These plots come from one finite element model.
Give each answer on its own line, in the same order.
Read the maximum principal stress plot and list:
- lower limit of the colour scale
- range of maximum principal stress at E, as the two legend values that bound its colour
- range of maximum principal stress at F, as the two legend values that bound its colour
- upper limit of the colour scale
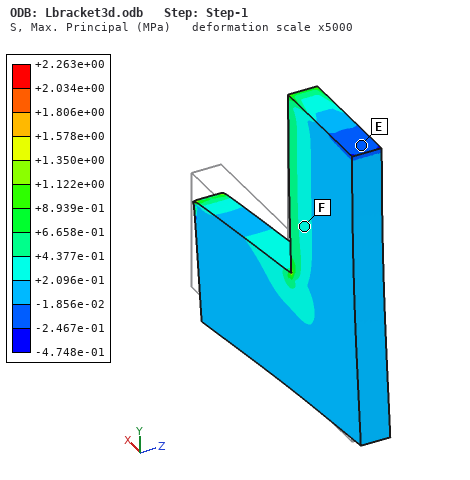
-4.748e-01 MPa
-2.467e-01 to -1.856e-02 MPa
+2.096e-01 to +4.377e-01 MPa
+2.263e+00 MPa
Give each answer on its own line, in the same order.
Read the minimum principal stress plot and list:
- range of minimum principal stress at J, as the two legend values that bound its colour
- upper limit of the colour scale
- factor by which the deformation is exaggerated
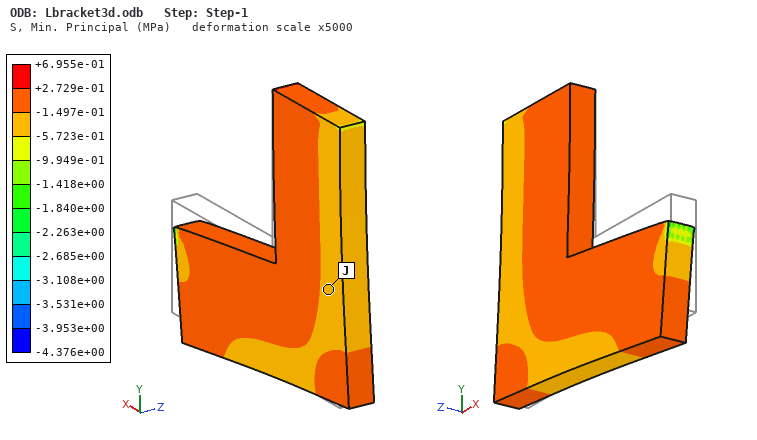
-5.723e-01 to -1.497e-01 MPa
+6.955e-01 MPa
5000
